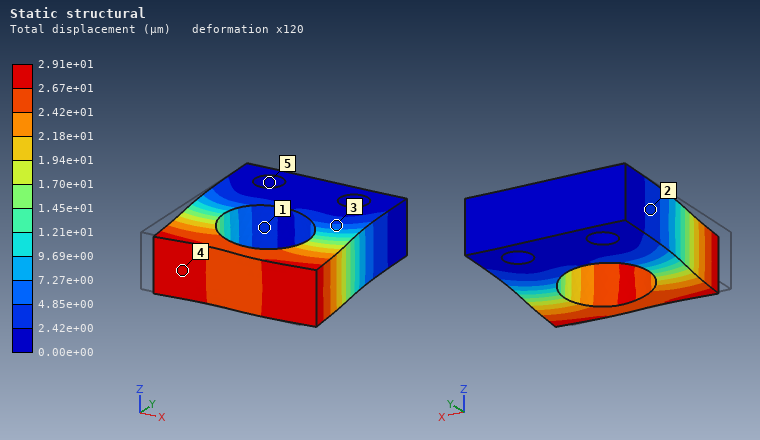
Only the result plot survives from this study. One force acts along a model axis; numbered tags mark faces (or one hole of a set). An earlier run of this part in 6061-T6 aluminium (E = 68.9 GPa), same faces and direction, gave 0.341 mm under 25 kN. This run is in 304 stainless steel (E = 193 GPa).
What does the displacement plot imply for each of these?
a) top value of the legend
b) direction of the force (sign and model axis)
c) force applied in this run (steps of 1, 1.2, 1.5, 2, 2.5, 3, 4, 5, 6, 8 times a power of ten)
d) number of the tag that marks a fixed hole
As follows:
2.91e+01 µm
+X
6 kN
5
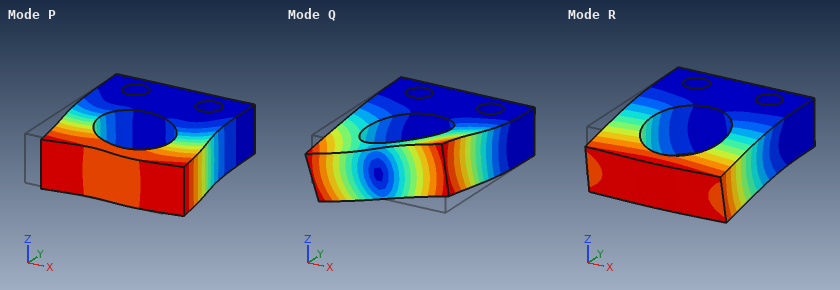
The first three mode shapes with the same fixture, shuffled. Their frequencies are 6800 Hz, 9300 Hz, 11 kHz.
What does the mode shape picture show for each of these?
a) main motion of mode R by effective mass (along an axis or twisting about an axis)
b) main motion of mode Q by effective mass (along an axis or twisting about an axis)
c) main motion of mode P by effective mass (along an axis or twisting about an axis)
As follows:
along Z
twisting about Y
along X
